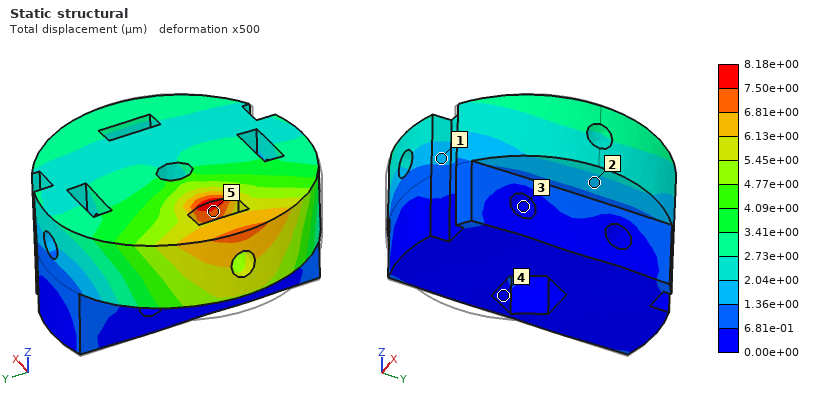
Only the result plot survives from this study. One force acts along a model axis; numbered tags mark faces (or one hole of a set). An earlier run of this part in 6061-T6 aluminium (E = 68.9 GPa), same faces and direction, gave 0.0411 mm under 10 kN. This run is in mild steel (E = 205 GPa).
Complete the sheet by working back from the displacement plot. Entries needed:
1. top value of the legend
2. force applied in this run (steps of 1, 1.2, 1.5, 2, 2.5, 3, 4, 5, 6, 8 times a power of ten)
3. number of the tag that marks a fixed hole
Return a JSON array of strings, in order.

["8.18e+00 µm", "6 kN", "3"]
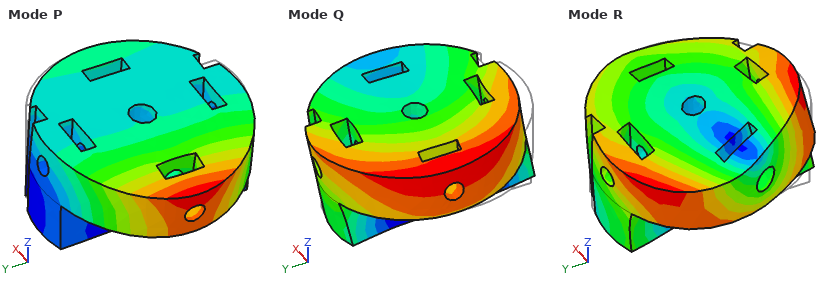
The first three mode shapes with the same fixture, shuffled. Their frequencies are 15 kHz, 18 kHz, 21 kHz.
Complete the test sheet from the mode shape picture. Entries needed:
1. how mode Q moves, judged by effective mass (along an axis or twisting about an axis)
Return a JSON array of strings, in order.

["along Y"]
